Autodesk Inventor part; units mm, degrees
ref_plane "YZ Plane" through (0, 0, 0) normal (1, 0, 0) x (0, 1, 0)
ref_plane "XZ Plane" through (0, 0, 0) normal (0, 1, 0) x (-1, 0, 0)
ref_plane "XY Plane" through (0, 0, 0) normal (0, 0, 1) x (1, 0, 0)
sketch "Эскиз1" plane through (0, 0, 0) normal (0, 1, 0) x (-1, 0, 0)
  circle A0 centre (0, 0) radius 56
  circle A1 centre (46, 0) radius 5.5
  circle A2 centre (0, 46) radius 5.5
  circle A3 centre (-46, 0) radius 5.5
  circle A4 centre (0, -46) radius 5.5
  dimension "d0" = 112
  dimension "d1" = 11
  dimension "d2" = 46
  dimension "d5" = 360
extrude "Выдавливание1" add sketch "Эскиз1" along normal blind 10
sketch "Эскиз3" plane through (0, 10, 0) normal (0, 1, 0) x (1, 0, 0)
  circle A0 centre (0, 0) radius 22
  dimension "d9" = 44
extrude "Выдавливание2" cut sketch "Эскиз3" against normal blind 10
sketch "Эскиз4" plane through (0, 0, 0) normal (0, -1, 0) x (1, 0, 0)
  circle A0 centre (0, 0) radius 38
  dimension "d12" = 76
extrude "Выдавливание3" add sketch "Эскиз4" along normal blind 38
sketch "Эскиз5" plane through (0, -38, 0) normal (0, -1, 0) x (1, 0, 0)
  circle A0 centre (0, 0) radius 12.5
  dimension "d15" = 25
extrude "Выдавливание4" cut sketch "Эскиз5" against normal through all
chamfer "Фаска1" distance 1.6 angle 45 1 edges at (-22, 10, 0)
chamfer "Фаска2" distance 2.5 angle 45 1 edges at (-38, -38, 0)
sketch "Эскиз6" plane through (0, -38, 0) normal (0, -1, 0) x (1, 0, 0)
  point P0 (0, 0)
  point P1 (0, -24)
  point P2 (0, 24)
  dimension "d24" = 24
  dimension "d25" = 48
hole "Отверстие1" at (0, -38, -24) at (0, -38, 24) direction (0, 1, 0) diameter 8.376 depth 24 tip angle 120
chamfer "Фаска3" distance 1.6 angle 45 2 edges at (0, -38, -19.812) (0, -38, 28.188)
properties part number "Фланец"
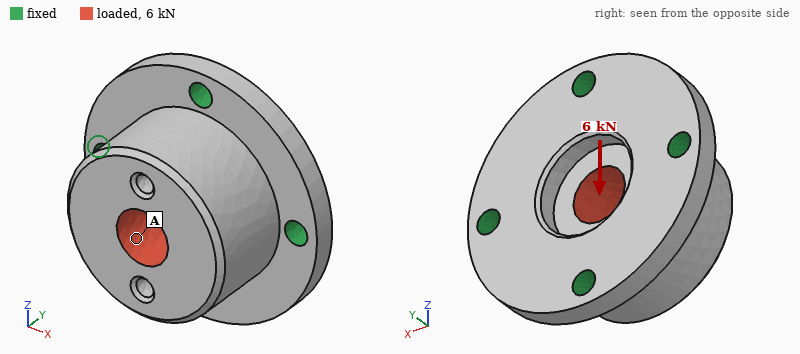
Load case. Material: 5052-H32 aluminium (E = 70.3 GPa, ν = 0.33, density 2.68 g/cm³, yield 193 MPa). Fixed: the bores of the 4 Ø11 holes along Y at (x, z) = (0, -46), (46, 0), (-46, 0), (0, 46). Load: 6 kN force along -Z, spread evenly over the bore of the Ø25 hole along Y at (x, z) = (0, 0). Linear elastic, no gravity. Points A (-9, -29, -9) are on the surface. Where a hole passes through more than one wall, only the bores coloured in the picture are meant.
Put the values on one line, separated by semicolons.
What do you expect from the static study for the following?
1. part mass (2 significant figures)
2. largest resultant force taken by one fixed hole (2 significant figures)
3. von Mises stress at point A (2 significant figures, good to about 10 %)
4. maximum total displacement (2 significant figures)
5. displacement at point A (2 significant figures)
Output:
620 g; 2.6 kN; 3.6 MPa; 7.1 µm; 5.9 µm
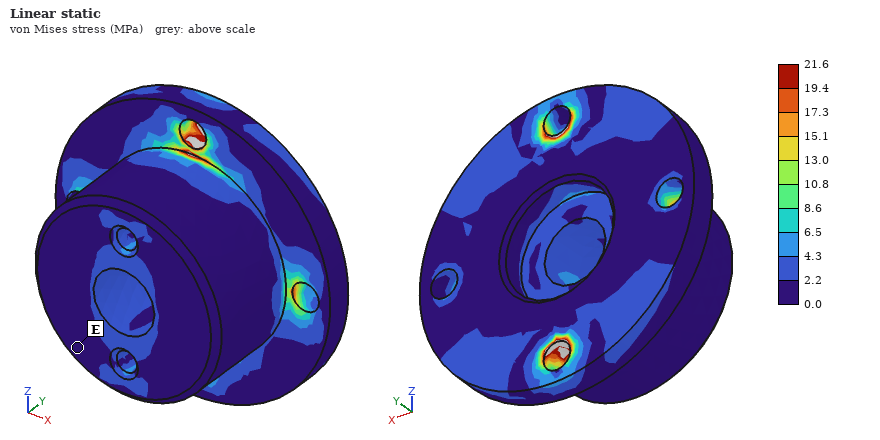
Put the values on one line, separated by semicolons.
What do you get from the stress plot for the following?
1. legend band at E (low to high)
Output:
0.0 to 2.2 MPa
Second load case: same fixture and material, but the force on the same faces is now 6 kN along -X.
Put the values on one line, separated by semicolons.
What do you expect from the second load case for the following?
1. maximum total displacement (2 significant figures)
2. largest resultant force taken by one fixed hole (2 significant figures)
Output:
7.1 µm; 2.6 kN
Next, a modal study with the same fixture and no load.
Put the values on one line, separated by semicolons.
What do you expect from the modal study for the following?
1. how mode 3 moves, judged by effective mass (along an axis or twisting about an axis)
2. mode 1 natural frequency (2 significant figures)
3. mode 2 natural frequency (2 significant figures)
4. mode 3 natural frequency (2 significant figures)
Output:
along Y; 7900 Hz; 7900 Hz; 9100 Hz
